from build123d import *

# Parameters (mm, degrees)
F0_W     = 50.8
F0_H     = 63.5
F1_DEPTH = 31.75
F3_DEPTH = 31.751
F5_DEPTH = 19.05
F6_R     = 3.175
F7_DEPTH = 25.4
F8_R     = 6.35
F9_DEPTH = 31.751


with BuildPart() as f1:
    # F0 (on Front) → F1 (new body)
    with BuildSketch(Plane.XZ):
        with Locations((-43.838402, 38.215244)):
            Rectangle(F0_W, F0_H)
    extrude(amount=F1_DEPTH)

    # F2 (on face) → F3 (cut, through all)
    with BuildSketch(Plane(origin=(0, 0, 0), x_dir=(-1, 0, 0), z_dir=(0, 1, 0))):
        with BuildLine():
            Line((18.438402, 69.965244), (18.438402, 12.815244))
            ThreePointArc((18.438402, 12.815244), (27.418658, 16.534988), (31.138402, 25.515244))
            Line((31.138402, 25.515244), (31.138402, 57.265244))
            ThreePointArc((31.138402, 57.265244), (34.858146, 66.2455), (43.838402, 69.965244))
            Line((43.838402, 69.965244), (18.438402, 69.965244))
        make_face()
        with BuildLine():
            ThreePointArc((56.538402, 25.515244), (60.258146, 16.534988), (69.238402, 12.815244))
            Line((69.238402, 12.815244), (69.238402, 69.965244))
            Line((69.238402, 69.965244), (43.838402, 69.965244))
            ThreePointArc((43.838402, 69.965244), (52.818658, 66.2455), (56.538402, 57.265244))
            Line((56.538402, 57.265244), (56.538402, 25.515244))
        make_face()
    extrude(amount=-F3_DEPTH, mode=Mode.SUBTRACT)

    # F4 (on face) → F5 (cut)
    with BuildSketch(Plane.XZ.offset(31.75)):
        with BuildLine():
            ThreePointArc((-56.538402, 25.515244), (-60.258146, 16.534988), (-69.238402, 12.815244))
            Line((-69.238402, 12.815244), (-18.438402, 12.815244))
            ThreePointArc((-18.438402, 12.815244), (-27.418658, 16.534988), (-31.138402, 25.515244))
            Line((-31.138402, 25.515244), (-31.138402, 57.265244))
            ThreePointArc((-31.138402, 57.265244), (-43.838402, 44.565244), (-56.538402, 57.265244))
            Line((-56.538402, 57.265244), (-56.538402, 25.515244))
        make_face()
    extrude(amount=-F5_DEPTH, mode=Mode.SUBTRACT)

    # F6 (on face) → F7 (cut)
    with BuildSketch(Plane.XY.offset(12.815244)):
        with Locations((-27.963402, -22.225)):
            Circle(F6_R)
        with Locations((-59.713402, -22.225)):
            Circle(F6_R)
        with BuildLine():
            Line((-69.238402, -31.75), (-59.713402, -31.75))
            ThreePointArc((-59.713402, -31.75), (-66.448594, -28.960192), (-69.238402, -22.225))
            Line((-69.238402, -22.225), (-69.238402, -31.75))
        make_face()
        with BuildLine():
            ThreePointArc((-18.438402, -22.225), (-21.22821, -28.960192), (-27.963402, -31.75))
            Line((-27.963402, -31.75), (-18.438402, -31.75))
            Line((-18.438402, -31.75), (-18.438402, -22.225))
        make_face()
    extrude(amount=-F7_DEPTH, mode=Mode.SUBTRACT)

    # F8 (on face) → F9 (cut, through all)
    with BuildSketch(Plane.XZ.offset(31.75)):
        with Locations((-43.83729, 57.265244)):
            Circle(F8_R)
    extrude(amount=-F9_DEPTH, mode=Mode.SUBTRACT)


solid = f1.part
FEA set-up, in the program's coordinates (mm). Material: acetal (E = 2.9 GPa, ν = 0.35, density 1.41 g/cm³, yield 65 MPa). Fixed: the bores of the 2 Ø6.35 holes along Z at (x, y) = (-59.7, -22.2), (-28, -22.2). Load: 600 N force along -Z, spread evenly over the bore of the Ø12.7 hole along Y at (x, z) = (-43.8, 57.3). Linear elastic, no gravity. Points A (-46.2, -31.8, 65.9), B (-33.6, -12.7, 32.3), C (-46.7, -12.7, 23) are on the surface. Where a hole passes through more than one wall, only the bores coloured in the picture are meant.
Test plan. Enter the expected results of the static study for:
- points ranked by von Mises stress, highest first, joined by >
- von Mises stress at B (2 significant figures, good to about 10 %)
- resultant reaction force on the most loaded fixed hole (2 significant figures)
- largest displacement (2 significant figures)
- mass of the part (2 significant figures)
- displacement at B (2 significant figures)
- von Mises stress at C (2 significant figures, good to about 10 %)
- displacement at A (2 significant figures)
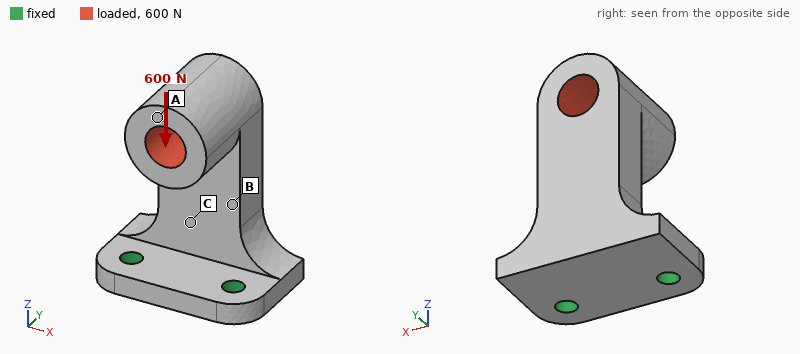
B > C > A
10 MPa
300 N
0.88 mm
47 g
0.15 mm
8.3 MPa
0.82 mm
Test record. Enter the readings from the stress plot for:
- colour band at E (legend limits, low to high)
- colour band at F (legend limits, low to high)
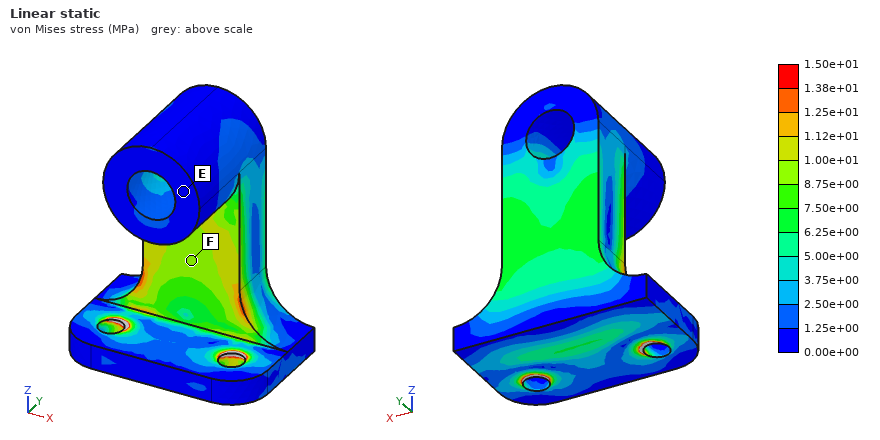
0.00e+00 to 1.25e+00 MPa
8.75e+00 to 1.00e+01 MPa
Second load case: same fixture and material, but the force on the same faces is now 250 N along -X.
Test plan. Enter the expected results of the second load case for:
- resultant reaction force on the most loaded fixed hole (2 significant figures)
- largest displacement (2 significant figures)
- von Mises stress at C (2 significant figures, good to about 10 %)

380 N
0.88 mm
6.4 MPa
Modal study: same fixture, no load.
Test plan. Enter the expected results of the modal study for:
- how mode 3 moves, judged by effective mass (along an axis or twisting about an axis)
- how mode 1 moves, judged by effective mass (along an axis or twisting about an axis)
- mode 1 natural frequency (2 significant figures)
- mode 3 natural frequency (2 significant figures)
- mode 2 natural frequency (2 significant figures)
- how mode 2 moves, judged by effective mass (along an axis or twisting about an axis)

along Z
along Y
320 Hz
1500 Hz
720 Hz
along X
